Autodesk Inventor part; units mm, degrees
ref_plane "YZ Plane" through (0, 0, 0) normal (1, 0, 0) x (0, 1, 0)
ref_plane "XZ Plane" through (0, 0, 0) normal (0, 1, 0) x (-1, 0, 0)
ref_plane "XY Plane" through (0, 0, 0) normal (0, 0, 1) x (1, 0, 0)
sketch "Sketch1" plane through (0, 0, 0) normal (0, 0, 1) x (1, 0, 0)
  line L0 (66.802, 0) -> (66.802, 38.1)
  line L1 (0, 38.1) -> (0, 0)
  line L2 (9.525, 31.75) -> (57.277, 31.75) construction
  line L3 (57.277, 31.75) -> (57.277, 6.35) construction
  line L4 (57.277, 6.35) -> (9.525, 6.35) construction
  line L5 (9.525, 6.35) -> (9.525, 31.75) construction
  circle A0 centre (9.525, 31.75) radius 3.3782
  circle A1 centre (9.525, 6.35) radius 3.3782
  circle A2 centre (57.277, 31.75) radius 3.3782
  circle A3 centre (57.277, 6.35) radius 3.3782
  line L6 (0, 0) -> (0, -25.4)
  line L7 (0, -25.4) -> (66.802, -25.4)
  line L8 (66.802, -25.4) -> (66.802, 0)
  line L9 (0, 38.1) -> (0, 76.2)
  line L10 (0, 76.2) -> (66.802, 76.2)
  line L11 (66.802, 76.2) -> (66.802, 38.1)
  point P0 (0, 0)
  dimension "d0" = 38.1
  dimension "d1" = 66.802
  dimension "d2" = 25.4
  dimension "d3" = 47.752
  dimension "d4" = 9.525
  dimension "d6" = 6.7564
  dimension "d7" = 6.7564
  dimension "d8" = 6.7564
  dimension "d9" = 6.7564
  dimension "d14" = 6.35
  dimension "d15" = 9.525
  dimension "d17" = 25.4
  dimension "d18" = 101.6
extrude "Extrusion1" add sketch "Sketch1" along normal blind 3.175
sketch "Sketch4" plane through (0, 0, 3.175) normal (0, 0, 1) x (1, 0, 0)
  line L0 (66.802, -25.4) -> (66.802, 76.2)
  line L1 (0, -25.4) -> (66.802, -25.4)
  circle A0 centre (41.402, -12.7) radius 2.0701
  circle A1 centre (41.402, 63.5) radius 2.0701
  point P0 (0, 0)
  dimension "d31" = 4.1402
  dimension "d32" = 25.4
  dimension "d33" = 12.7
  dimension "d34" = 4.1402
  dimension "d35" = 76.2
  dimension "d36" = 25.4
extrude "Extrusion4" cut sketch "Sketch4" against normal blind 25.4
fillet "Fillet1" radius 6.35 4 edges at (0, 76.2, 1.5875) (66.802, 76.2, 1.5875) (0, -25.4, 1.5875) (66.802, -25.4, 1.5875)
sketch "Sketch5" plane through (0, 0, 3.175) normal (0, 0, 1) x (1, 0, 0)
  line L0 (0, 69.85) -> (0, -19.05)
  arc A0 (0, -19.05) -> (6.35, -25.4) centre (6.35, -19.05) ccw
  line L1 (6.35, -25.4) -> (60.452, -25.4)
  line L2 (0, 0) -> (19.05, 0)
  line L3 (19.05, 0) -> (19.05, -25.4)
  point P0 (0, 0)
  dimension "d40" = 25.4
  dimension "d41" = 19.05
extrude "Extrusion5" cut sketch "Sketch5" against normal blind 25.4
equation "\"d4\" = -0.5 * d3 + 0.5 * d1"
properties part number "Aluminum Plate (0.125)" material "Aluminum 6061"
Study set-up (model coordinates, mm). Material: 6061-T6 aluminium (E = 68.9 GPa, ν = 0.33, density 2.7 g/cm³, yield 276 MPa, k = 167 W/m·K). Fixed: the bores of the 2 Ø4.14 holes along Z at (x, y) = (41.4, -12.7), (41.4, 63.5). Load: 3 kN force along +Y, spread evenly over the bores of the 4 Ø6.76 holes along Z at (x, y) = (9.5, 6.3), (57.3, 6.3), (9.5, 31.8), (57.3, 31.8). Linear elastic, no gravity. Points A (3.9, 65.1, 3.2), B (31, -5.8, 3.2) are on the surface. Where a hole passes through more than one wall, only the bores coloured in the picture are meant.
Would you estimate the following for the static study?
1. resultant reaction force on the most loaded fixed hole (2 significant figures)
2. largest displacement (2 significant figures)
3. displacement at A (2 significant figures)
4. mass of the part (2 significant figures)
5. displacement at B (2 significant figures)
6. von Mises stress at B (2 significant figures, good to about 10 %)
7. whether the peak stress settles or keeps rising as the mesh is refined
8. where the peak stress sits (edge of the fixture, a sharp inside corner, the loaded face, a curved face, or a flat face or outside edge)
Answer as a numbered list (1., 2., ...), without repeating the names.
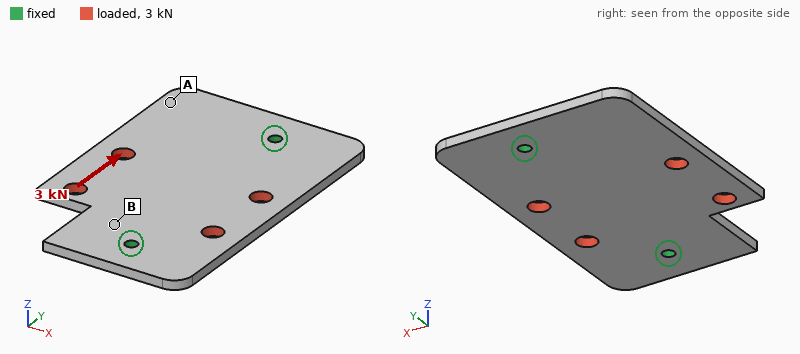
1. 1.6 kN
2. 18 µm
3. 12 µm
4. 52 g
5. 4.7 µm
6. 17 MPa
7. keeps rising
8. edge of the fixture
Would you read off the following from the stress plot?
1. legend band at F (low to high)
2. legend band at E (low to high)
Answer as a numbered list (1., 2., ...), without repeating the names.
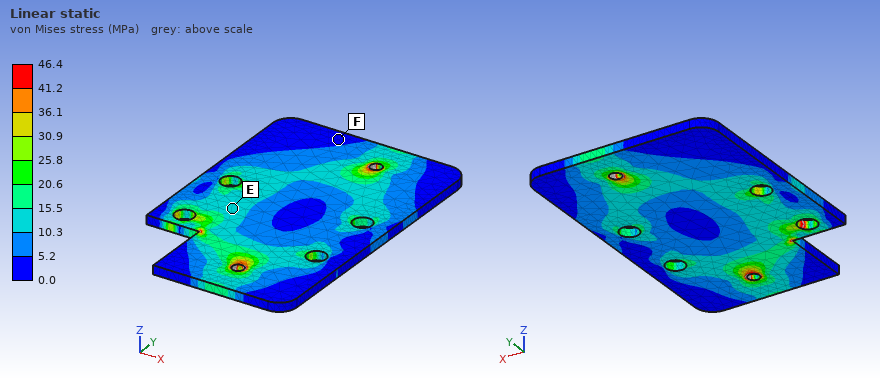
1. 0.0 to 5.2 MPa
2. 10.3 to 15.5 MPa
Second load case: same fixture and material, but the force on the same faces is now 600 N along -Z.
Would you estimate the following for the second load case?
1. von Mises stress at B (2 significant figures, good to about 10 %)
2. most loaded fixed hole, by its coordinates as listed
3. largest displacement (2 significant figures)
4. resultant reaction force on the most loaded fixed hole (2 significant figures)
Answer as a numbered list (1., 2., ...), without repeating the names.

1. 46 MPa
2. (41.4, -12.7)
3. 0.53 mm
4. 360 N
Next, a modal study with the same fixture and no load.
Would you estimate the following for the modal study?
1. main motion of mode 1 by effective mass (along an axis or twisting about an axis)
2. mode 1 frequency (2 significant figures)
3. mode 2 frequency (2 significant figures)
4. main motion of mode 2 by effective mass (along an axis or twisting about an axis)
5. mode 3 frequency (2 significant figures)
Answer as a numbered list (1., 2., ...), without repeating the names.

1. along Z
2. 1200 Hz
3. 2200 Hz
4. along Z
5. 2500 Hz
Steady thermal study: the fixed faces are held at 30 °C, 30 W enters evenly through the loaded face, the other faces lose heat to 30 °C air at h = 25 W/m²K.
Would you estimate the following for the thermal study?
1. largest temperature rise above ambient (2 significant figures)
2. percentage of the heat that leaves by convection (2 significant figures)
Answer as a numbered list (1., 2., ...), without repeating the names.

1. 29 K
2. 14 %
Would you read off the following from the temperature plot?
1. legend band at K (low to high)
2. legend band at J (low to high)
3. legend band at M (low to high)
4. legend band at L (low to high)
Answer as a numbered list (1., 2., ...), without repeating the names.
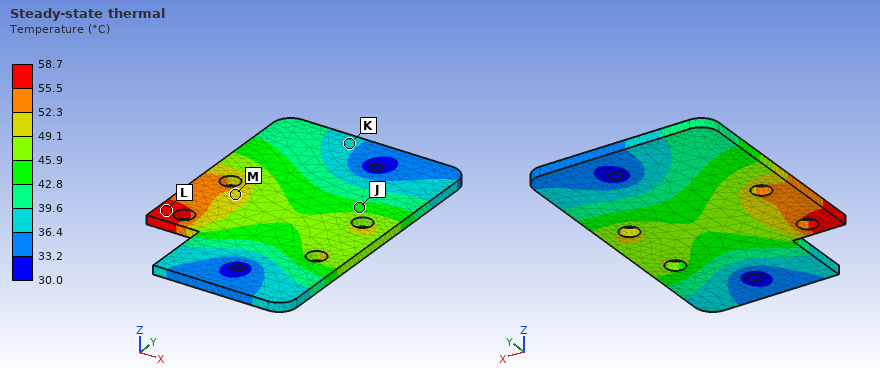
1. 36.4 to 39.6 °C
2. 42.8 to 45.9 °C
3. 49.1 to 52.3 °C
4. 55.5 to 58.7 °C
